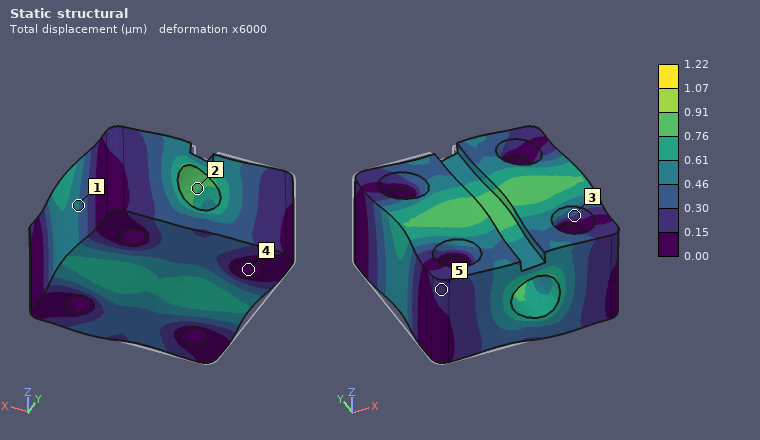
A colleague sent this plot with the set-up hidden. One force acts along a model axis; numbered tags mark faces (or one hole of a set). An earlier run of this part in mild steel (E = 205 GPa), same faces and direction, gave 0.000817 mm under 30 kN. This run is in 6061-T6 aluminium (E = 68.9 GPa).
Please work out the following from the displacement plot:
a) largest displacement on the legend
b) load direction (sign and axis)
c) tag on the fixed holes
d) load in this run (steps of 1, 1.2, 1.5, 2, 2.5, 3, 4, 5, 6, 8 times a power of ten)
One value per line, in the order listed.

1.22 µm
+X
4
15 kN
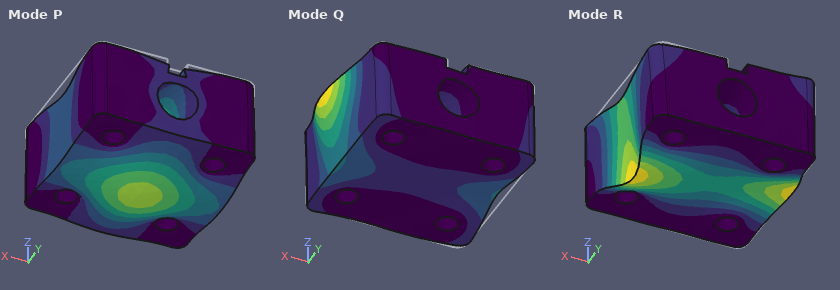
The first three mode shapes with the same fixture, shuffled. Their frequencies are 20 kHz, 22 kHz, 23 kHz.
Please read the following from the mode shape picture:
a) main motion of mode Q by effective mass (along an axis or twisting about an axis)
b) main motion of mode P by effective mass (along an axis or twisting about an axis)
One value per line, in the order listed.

along X
along Z
